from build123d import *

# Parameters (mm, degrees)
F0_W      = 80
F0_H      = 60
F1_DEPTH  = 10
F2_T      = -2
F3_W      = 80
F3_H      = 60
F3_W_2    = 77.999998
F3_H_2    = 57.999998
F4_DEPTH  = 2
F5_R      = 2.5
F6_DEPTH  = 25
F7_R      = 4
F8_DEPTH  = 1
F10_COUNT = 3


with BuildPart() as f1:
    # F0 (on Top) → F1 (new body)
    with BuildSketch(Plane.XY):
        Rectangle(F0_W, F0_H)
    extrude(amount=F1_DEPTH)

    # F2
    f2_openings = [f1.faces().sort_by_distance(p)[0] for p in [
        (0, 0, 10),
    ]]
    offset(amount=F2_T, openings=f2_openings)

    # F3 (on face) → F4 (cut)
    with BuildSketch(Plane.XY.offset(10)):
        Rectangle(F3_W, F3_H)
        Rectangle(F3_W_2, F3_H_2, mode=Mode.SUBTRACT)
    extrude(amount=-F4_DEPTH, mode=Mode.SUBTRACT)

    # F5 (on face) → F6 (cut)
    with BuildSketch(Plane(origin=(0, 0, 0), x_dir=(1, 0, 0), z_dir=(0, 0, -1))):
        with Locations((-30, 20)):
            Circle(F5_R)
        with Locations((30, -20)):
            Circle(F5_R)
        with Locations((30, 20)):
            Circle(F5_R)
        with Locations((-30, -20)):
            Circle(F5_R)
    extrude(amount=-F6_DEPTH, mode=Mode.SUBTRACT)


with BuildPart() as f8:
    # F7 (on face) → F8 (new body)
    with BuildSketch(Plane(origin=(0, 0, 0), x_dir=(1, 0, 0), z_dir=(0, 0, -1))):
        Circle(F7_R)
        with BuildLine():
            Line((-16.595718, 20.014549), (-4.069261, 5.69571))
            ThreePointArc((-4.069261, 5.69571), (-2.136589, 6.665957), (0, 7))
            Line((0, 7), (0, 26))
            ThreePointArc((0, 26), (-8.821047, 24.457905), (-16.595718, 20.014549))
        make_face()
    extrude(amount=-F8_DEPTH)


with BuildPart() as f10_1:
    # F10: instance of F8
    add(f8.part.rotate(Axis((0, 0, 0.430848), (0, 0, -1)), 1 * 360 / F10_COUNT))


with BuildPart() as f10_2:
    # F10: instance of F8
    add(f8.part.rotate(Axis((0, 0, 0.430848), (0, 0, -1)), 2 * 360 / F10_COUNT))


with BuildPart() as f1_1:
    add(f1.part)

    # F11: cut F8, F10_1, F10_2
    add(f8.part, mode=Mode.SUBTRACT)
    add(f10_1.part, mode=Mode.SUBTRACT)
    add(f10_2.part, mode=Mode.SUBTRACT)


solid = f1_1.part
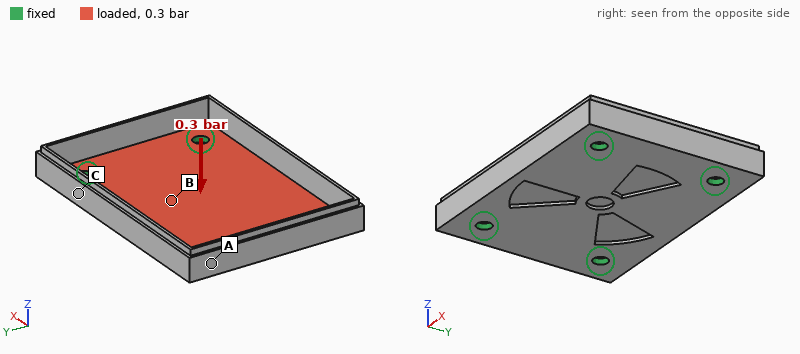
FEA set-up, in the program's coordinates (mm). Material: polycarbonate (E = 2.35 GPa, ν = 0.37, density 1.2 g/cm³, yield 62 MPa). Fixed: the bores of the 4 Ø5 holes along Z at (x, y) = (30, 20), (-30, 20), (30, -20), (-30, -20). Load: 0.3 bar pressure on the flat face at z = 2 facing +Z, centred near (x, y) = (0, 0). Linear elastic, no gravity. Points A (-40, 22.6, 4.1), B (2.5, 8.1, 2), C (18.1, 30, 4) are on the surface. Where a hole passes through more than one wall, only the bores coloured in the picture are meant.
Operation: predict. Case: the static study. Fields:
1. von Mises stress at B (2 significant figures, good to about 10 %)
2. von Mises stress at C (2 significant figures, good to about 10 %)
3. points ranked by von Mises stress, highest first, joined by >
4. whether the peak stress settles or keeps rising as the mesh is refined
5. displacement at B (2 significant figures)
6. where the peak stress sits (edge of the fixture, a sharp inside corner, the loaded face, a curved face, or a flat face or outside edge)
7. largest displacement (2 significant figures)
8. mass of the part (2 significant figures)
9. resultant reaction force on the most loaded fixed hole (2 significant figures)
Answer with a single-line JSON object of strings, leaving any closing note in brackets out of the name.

{"von Mises stress at B": "4.4 MPa", "von Mises stress at C": "2.2 MPa", "points ranked by von Mises stress, highest first, joined by >": "B > C > A", "whether the peak stress settles or keeps rising as the mesh is refined": "keeps rising", "displacement at B": "0.61 mm", "where the peak stress sits": "edge of the fixture", "largest displacement": "0.72 mm", "mass of the part": "15 g", "resultant reaction force on the most loaded fixed hole": "41 N"}
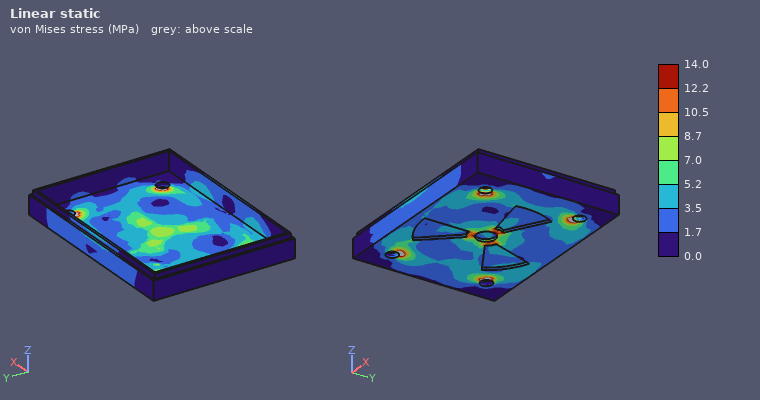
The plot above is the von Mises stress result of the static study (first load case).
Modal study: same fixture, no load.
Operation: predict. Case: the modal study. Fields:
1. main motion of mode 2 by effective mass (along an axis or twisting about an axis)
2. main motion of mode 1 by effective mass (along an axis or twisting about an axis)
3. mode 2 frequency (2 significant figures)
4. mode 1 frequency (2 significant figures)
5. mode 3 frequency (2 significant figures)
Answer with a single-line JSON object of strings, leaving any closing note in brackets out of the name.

{"main motion of mode 2 by effective mass": "twisting about X", "main motion of mode 1 by effective mass": "along Z", "mode 2 frequency": "1600 Hz", "mode 1 frequency": "930 Hz", "mode 3 frequency": "1700 Hz"}
